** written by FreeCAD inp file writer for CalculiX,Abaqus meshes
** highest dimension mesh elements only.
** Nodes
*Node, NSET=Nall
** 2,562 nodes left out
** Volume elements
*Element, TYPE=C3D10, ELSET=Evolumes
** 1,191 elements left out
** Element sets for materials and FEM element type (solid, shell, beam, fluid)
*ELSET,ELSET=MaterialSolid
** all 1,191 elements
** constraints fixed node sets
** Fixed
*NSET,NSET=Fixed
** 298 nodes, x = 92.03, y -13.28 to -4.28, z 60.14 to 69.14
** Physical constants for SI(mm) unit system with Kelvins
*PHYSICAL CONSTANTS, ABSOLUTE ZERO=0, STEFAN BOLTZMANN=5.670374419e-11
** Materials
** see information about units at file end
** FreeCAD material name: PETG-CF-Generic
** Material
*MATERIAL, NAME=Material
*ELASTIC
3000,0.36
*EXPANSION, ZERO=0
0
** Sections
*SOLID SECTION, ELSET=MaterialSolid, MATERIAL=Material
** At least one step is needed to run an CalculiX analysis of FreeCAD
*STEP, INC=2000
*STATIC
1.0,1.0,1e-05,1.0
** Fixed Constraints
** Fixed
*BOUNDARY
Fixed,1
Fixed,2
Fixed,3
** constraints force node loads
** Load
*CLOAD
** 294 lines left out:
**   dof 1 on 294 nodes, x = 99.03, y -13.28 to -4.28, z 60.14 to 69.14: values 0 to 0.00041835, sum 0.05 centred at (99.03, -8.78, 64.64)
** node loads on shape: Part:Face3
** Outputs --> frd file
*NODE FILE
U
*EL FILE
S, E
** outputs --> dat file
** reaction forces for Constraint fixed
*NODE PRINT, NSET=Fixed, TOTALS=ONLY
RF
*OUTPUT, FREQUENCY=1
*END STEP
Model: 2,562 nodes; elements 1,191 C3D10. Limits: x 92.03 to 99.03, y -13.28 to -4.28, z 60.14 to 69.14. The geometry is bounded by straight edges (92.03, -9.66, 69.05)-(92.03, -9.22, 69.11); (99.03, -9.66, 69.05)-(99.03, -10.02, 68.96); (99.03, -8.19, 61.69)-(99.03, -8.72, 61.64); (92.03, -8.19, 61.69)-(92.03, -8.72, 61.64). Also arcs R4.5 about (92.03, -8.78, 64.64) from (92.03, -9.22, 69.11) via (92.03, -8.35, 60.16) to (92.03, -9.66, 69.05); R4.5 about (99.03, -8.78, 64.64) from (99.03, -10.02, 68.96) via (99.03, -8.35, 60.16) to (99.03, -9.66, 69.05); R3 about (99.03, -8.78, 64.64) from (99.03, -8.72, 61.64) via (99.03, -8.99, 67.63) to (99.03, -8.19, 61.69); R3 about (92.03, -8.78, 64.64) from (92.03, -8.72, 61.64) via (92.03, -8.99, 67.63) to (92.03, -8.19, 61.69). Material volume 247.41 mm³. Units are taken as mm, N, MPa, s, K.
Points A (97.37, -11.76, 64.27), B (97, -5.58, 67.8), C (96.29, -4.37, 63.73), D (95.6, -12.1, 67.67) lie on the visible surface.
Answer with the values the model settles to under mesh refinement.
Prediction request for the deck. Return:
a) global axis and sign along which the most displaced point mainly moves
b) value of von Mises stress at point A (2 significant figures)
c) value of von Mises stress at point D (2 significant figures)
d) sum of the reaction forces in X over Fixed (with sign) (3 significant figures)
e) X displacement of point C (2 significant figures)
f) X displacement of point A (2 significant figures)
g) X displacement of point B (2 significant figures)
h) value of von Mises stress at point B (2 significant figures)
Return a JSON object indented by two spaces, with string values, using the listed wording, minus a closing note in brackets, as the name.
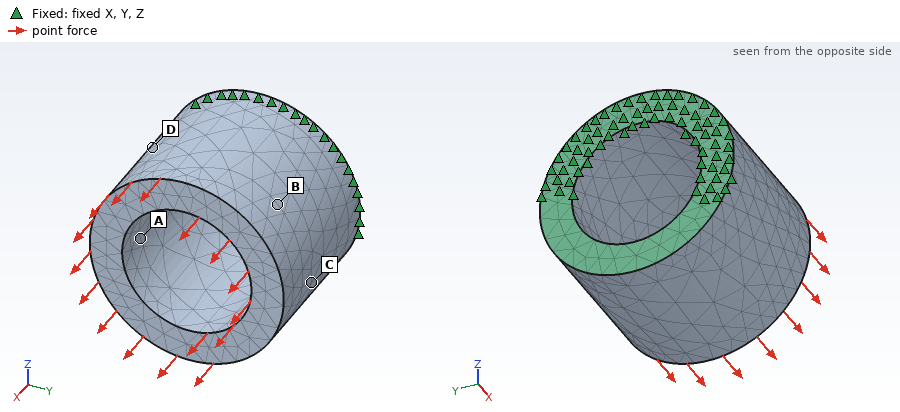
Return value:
{
  "global axis and sign along which the most displaced point mainly moves": "+X",
  "value of von Mises stress at point A": "0.0015 MPa",
  "value of von Mises stress at point D": "0.0013 MPa",
  "sum of the reaction forces in X over Fixed (with sign)": "-0.0500 N",
  "X displacement of point C": "1.9e-06 mm",
  "X displacement of point A": "2.4e-06 mm",
  "X displacement of point B": "2.2e-06 mm",
  "value of von Mises stress at point B": "0.0014 MPa"
}
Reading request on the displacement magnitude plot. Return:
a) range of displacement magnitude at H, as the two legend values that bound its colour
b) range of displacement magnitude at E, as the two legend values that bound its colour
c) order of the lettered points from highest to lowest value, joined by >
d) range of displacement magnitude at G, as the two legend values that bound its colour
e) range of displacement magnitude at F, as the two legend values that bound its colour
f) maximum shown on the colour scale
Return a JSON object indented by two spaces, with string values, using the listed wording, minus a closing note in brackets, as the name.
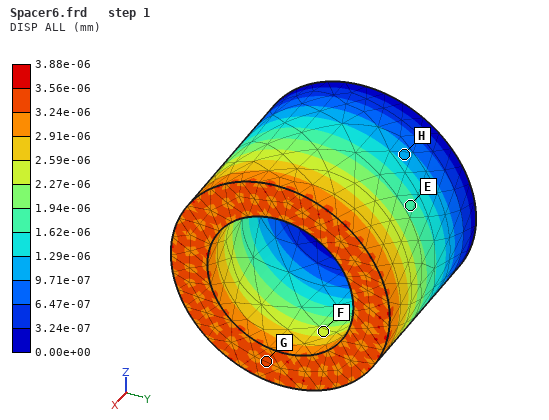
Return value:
{
  "range of displacement magnitude at H, as the two legend values that bound its colour": "9.71e-07 to 1.29e-06 mm",
  "range of displacement magnitude at E, as the two legend values that bound its colour": "1.62e-06 to 1.94e-06 mm",
  "order of the lettered points from highest to lowest value, joined by >": "G > F > E > H",
  "range of displacement magnitude at G, as the two legend values that bound its colour": "3.24e-06 to 3.56e-06 mm",
  "range of displacement magnitude at F, as the two legend values that bound its colour": "2.27e-06 to 2.59e-06 mm",
  "maximum shown on the colour scale": "3.88e-06 mm"
}
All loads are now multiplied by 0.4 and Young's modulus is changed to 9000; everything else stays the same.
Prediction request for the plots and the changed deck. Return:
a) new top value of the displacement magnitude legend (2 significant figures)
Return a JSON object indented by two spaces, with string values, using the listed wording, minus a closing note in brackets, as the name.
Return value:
{
  "new top value of the displacement magnitude legend": "5.2e-07 mm"
}
